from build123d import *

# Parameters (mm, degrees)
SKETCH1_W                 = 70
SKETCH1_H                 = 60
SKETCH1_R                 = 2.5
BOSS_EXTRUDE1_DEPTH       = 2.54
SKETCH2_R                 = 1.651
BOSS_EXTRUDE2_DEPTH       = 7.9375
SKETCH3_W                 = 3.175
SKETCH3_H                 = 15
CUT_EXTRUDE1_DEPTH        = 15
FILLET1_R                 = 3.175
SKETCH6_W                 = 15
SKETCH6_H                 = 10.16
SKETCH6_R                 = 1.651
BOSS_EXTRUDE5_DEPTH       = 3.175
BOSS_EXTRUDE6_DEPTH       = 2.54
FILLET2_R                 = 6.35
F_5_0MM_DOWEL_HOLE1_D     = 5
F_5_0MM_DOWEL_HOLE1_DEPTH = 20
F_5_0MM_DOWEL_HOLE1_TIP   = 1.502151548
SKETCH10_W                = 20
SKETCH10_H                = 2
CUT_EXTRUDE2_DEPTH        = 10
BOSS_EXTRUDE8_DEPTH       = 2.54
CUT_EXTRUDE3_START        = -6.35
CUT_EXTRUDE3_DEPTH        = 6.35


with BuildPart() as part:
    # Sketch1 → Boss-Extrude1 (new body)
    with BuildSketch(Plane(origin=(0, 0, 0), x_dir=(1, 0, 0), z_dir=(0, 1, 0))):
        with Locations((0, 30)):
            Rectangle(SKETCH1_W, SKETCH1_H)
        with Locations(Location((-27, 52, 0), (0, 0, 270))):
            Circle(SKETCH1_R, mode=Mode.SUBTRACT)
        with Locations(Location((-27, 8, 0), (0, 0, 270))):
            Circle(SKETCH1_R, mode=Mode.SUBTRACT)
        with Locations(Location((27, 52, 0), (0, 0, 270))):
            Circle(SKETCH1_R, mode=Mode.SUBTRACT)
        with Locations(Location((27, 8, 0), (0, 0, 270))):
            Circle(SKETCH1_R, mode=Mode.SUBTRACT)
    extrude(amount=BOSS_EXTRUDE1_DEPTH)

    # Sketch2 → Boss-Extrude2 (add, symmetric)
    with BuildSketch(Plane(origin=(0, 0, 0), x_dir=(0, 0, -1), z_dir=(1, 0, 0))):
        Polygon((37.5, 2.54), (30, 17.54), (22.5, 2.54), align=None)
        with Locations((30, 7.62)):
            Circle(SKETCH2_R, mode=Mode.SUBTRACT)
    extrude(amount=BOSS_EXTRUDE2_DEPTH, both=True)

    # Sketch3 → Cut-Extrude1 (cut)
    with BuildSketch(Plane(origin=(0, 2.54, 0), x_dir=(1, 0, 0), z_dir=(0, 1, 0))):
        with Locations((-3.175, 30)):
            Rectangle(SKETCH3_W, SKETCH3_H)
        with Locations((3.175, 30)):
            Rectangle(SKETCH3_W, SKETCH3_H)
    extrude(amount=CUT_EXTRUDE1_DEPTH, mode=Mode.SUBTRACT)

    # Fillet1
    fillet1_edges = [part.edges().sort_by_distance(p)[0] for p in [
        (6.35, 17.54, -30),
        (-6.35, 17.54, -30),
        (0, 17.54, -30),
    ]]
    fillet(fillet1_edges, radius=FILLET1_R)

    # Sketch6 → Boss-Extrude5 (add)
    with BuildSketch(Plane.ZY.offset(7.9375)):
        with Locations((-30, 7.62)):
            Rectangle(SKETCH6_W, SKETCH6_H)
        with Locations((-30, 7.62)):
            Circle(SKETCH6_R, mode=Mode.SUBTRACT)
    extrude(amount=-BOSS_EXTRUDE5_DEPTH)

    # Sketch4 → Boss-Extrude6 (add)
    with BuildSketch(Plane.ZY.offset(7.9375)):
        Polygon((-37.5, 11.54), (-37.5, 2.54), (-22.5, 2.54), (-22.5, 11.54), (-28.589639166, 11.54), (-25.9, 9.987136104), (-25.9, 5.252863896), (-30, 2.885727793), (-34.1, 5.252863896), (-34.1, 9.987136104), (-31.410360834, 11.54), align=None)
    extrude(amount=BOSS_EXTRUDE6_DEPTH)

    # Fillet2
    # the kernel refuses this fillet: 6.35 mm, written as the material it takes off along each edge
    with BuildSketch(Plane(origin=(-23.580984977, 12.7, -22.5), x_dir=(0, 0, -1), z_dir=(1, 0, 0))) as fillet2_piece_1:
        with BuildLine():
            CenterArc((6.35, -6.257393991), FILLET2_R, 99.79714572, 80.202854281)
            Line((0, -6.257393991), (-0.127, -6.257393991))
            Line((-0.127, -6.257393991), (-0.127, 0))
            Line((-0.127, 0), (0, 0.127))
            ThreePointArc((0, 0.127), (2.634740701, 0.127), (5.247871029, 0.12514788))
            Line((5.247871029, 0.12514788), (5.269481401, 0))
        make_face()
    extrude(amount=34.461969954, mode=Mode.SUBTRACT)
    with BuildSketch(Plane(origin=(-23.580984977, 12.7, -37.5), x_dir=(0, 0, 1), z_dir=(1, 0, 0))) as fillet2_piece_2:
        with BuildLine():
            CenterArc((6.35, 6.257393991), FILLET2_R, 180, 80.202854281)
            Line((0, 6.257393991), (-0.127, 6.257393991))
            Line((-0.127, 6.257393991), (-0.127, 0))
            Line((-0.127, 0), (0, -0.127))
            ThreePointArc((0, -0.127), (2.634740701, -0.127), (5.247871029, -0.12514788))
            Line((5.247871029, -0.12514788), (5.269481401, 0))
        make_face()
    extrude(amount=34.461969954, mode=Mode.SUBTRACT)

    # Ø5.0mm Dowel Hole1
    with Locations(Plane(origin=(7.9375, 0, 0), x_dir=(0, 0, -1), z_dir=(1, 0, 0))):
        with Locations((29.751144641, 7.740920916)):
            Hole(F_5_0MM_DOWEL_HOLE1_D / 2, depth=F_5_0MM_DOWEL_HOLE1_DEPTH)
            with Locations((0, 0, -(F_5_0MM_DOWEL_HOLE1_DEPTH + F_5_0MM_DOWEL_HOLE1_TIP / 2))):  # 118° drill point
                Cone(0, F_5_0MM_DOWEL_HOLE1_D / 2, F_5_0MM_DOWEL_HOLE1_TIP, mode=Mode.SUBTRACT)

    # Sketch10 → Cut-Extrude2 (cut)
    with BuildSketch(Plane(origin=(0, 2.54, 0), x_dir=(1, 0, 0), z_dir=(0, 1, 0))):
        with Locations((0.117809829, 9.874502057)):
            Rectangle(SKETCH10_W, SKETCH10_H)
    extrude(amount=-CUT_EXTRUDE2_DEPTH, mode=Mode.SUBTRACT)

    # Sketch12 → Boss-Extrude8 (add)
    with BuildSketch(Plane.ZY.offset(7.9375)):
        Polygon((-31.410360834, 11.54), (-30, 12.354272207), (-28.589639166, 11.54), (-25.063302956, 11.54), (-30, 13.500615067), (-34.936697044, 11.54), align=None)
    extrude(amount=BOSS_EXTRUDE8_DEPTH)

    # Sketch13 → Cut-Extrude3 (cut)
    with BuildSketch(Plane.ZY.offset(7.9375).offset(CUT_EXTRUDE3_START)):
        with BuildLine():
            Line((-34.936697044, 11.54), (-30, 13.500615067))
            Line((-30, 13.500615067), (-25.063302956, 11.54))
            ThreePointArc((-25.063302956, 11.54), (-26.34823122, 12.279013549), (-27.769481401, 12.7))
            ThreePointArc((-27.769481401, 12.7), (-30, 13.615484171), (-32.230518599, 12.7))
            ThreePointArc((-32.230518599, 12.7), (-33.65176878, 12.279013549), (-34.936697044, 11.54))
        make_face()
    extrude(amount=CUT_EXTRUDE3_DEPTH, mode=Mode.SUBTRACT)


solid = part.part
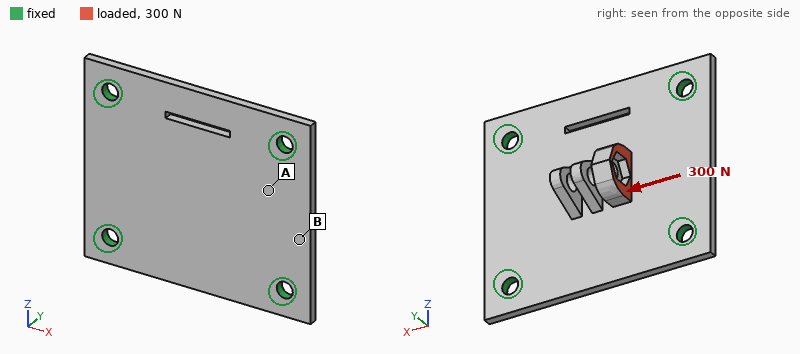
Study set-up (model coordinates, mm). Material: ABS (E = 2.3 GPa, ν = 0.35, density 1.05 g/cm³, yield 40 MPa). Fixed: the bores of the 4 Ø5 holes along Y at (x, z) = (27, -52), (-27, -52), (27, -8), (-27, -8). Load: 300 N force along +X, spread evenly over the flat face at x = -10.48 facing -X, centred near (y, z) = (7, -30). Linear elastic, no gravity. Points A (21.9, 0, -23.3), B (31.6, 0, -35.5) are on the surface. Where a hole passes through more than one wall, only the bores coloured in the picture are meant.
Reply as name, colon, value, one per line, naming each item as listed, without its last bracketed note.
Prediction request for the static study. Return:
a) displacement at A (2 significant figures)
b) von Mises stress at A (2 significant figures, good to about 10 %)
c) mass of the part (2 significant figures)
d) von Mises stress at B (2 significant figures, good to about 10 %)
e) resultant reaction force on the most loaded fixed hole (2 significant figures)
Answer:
displacement at A: 0.14 mm
von Mises stress at A: 3.1 MPa
mass of the part: 12 g
von Mises stress at B: 2.0 MPa
resultant reaction force on the most loaded fixed hole: 95 N
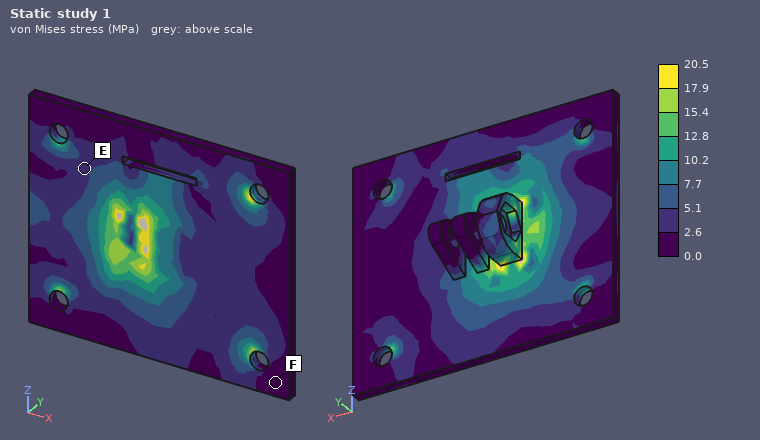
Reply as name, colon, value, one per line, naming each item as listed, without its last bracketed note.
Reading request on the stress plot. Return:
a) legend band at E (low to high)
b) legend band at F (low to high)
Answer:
legend band at E: 2.6 to 5.1 MPa
legend band at F: 0.0 to 2.6 MPa
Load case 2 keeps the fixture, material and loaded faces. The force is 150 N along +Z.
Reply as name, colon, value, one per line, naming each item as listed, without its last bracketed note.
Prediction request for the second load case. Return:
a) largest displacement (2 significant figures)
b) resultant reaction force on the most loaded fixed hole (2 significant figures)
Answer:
largest displacement: 0.29 mm
resultant reaction force on the most loaded fixed hole: 57 N
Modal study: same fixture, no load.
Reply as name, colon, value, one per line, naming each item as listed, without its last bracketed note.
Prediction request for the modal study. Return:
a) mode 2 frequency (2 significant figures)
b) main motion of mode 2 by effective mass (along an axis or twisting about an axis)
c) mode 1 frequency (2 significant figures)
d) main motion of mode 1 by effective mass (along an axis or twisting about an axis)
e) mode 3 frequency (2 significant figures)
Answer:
mode 2 frequency: 1600 Hz
main motion of mode 2 by effective mass: twisting about X
mode 1 frequency: 1000 Hz
main motion of mode 1 by effective mass: along Y
mode 3 frequency: 2100 Hz
